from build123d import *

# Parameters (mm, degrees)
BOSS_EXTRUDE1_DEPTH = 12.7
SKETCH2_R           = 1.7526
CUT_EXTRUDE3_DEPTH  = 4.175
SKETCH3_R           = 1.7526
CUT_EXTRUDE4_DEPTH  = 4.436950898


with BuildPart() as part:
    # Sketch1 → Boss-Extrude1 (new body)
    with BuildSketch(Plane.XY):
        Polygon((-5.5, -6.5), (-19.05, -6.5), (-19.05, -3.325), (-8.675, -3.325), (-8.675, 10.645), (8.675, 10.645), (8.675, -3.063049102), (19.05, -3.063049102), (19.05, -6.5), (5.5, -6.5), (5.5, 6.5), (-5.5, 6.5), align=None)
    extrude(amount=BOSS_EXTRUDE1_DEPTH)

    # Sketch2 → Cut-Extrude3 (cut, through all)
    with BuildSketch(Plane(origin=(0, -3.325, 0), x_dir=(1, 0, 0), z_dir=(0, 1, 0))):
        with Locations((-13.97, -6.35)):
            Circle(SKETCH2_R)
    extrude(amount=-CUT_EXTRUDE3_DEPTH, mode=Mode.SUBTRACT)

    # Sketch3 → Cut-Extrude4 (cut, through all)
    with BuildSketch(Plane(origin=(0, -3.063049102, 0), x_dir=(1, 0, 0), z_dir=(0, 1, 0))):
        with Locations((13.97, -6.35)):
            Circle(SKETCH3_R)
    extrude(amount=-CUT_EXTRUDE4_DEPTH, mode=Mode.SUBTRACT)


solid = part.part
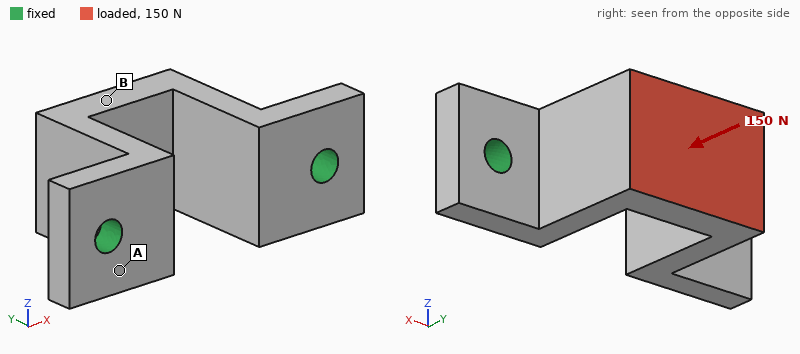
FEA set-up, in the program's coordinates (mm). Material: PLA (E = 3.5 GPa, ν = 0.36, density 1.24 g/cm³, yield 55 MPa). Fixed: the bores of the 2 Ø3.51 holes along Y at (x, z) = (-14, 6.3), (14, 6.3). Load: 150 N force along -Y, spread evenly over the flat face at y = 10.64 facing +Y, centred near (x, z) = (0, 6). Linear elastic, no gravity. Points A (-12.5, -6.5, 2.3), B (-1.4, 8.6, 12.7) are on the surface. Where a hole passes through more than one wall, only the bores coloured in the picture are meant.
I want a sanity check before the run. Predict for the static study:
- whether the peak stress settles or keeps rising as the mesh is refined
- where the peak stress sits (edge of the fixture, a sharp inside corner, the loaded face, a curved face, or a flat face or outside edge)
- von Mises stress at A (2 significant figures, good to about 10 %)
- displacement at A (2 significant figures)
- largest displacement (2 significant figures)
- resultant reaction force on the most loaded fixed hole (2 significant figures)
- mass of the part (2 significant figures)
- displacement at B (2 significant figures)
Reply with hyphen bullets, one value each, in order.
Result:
- keeps rising
- edge of the fixture
- 4.2 MPa
- 9.1 µm
- 42 µm
- 79 N
- 3.4 g
- 42 µm
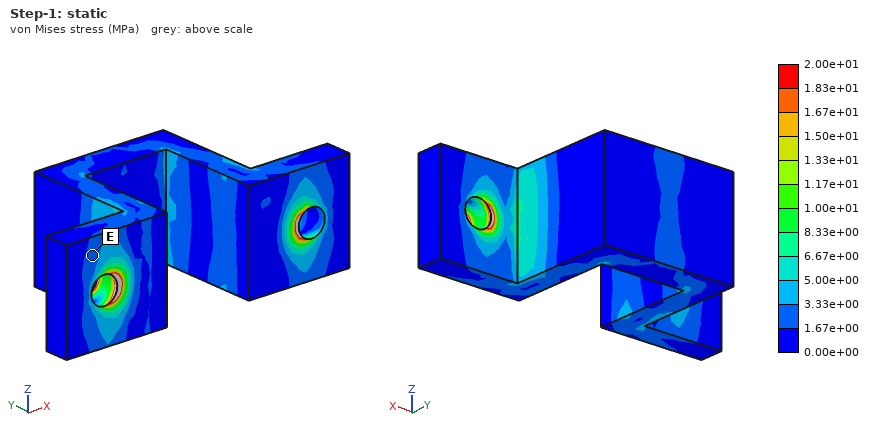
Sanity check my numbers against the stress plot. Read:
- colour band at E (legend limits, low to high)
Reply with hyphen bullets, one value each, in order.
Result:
- 1.67e+00 to 3.33e+00 MPa
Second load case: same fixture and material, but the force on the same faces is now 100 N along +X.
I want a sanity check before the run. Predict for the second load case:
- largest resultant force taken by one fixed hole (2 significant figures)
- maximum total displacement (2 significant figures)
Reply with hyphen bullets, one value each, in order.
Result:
- 82 N
- 0.12 mm
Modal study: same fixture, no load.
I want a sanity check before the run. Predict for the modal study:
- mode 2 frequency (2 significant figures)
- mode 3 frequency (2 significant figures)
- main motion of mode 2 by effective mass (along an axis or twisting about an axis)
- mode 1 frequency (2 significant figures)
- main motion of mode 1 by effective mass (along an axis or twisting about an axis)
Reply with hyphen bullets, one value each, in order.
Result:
- 3900 Hz
- 5400 Hz
- along X
- 2400 Hz
- along Z
